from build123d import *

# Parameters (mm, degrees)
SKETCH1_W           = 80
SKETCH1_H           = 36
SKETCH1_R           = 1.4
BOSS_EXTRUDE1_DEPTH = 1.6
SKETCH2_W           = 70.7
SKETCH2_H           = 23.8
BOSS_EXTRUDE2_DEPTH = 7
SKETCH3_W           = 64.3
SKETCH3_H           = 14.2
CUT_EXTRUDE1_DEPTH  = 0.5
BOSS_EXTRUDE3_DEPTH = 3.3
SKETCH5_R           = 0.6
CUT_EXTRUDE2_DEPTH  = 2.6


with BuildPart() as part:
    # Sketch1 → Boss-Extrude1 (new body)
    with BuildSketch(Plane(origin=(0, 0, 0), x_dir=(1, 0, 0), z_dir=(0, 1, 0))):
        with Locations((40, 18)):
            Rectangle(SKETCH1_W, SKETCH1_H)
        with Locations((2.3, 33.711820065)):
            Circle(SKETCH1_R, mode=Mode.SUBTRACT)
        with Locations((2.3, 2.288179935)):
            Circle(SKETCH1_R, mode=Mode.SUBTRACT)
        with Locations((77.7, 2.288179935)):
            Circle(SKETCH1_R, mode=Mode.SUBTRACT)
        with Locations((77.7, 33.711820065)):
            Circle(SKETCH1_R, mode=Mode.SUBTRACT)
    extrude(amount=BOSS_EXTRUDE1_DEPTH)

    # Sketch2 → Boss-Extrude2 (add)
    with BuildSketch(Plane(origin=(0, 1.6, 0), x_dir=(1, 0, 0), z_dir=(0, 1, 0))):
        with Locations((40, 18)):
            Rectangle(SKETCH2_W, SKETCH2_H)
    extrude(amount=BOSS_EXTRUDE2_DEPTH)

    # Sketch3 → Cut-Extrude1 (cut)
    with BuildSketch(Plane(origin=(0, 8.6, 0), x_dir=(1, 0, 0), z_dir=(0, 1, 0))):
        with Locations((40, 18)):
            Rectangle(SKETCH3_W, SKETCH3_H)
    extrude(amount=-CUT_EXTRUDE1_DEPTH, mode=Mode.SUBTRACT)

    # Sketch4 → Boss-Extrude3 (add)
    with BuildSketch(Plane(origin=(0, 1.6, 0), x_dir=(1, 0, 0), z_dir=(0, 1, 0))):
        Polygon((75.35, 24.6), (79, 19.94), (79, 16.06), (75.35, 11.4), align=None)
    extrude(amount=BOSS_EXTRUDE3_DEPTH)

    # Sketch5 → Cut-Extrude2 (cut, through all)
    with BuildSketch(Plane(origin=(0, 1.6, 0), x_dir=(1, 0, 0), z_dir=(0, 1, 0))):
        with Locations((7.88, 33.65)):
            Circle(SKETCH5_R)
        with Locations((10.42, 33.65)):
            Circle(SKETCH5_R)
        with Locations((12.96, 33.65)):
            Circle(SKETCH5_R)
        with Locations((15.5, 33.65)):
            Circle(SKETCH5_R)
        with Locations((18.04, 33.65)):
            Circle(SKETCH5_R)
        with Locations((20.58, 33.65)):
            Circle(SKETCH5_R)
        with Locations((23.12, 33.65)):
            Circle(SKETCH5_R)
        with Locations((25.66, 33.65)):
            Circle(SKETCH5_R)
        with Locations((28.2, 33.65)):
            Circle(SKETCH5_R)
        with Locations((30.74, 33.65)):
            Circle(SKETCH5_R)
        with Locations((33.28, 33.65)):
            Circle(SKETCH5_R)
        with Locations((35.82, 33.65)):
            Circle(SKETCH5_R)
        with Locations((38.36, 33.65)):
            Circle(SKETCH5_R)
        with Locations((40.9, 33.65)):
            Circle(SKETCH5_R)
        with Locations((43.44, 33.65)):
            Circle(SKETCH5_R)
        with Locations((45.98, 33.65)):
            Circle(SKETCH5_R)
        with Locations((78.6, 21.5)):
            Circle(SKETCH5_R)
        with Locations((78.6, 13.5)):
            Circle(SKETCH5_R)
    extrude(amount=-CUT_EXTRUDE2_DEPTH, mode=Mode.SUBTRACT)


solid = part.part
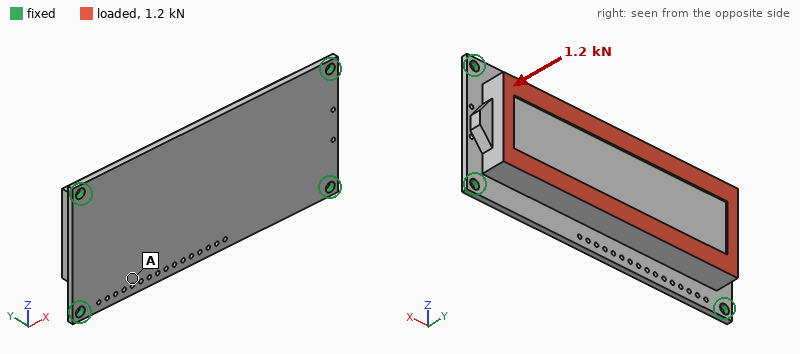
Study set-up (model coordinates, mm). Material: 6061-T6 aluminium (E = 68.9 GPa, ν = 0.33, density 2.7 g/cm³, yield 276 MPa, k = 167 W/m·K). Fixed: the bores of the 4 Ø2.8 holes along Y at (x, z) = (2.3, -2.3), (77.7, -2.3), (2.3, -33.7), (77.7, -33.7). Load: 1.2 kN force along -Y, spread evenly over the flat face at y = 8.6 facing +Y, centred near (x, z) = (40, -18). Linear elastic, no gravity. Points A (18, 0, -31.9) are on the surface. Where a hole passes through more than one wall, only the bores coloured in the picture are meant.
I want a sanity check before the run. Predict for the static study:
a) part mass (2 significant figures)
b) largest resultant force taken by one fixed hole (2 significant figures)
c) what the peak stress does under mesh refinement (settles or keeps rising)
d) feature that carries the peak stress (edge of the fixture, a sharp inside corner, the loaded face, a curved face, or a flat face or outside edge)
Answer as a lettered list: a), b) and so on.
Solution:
a) 43 g
b) 530 N
c) keeps rising
d) edge of the fixture
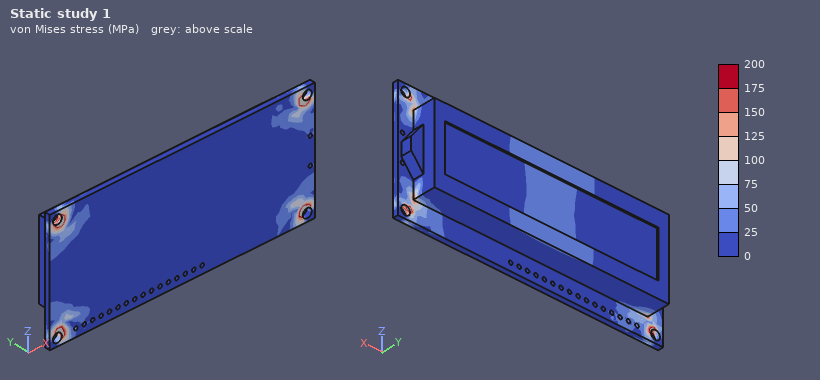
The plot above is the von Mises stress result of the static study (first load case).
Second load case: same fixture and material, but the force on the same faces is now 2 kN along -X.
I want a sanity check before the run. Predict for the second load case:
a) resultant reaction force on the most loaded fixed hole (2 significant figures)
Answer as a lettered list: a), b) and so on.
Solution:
a) 560 N
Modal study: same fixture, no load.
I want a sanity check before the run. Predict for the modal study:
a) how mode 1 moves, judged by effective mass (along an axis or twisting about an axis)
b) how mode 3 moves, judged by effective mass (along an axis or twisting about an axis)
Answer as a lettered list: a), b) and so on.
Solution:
a) along Y
b) twisting about Z
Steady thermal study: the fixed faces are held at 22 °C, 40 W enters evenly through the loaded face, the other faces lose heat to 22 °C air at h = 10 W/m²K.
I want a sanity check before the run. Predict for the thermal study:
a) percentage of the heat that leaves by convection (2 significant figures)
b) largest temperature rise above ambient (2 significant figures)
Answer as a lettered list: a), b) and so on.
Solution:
a) 4.5 %
b) 33 K
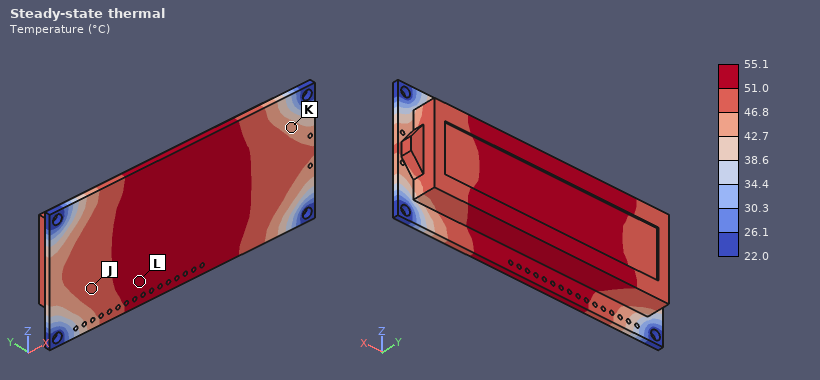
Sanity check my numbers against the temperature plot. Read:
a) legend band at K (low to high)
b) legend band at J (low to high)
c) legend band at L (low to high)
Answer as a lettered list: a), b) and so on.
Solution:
a) 42.7 to 46.8 °C
b) 46.8 to 51.0 °C
c) 51.0 to 55.1 °C
